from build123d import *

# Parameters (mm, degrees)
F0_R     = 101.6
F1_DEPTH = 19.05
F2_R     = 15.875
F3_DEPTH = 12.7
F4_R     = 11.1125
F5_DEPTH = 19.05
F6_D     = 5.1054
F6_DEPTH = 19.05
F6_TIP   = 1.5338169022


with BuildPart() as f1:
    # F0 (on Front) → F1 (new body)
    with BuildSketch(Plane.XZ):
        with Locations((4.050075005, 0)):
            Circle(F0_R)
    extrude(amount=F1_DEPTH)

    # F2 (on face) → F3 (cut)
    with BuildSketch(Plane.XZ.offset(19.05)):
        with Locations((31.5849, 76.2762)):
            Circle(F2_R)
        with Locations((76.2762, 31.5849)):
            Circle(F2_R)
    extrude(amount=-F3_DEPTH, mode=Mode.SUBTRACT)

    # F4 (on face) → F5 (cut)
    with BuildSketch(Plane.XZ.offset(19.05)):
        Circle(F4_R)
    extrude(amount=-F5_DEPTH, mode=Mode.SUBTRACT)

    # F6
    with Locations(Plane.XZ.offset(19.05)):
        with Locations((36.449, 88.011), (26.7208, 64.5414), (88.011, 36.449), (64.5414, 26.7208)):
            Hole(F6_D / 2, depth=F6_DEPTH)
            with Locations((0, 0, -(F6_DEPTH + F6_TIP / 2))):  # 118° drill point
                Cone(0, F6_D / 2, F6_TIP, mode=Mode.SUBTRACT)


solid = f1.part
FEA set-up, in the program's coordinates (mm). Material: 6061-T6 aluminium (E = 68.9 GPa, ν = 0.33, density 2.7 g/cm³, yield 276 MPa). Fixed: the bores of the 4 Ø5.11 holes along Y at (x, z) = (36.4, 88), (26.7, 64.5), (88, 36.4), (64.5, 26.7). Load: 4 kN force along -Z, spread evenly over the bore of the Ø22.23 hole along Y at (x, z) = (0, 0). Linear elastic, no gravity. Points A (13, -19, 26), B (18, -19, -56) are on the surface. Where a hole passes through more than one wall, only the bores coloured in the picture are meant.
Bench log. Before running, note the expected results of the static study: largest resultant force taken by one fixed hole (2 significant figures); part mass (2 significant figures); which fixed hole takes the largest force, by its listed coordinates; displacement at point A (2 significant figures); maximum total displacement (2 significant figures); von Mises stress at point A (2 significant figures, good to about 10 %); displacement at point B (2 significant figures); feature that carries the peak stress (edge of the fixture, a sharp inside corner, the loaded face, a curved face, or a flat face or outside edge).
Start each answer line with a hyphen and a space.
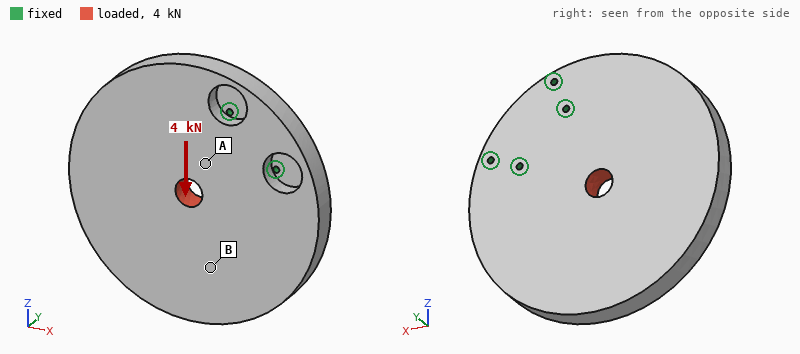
- 3.0 kN
- 1.6 kg
- (26.7, 64.5)
- 11 µm
- 35 µm
- 3.6 MPa
- 19 µm
- edge of the fixture
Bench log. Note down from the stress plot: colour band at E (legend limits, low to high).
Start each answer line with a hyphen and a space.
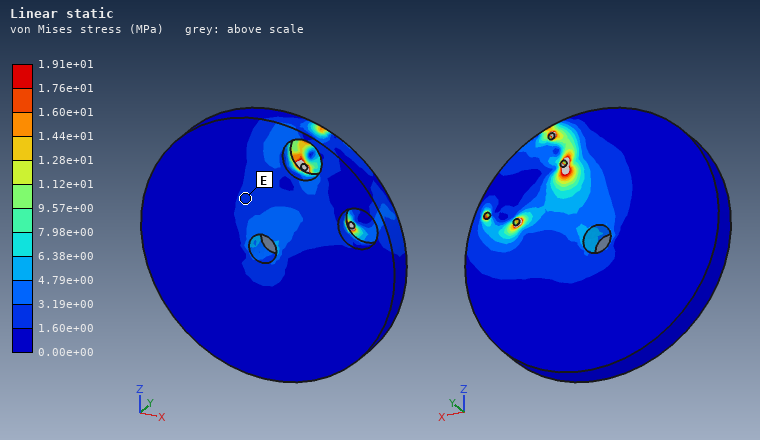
- 1.60e+00 to 3.19e+00 MPa
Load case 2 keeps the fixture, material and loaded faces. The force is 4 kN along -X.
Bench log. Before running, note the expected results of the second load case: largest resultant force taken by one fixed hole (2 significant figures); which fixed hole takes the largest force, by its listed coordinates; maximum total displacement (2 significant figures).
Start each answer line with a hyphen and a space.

- 3.0 kN
- (64.5, 26.7)
- 35 µm
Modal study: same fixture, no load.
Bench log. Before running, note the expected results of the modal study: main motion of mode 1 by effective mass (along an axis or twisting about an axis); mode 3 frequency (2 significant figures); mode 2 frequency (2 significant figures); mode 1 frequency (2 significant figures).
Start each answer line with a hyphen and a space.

- along Y
- 1600 Hz
- 910 Hz
- 420 Hz
